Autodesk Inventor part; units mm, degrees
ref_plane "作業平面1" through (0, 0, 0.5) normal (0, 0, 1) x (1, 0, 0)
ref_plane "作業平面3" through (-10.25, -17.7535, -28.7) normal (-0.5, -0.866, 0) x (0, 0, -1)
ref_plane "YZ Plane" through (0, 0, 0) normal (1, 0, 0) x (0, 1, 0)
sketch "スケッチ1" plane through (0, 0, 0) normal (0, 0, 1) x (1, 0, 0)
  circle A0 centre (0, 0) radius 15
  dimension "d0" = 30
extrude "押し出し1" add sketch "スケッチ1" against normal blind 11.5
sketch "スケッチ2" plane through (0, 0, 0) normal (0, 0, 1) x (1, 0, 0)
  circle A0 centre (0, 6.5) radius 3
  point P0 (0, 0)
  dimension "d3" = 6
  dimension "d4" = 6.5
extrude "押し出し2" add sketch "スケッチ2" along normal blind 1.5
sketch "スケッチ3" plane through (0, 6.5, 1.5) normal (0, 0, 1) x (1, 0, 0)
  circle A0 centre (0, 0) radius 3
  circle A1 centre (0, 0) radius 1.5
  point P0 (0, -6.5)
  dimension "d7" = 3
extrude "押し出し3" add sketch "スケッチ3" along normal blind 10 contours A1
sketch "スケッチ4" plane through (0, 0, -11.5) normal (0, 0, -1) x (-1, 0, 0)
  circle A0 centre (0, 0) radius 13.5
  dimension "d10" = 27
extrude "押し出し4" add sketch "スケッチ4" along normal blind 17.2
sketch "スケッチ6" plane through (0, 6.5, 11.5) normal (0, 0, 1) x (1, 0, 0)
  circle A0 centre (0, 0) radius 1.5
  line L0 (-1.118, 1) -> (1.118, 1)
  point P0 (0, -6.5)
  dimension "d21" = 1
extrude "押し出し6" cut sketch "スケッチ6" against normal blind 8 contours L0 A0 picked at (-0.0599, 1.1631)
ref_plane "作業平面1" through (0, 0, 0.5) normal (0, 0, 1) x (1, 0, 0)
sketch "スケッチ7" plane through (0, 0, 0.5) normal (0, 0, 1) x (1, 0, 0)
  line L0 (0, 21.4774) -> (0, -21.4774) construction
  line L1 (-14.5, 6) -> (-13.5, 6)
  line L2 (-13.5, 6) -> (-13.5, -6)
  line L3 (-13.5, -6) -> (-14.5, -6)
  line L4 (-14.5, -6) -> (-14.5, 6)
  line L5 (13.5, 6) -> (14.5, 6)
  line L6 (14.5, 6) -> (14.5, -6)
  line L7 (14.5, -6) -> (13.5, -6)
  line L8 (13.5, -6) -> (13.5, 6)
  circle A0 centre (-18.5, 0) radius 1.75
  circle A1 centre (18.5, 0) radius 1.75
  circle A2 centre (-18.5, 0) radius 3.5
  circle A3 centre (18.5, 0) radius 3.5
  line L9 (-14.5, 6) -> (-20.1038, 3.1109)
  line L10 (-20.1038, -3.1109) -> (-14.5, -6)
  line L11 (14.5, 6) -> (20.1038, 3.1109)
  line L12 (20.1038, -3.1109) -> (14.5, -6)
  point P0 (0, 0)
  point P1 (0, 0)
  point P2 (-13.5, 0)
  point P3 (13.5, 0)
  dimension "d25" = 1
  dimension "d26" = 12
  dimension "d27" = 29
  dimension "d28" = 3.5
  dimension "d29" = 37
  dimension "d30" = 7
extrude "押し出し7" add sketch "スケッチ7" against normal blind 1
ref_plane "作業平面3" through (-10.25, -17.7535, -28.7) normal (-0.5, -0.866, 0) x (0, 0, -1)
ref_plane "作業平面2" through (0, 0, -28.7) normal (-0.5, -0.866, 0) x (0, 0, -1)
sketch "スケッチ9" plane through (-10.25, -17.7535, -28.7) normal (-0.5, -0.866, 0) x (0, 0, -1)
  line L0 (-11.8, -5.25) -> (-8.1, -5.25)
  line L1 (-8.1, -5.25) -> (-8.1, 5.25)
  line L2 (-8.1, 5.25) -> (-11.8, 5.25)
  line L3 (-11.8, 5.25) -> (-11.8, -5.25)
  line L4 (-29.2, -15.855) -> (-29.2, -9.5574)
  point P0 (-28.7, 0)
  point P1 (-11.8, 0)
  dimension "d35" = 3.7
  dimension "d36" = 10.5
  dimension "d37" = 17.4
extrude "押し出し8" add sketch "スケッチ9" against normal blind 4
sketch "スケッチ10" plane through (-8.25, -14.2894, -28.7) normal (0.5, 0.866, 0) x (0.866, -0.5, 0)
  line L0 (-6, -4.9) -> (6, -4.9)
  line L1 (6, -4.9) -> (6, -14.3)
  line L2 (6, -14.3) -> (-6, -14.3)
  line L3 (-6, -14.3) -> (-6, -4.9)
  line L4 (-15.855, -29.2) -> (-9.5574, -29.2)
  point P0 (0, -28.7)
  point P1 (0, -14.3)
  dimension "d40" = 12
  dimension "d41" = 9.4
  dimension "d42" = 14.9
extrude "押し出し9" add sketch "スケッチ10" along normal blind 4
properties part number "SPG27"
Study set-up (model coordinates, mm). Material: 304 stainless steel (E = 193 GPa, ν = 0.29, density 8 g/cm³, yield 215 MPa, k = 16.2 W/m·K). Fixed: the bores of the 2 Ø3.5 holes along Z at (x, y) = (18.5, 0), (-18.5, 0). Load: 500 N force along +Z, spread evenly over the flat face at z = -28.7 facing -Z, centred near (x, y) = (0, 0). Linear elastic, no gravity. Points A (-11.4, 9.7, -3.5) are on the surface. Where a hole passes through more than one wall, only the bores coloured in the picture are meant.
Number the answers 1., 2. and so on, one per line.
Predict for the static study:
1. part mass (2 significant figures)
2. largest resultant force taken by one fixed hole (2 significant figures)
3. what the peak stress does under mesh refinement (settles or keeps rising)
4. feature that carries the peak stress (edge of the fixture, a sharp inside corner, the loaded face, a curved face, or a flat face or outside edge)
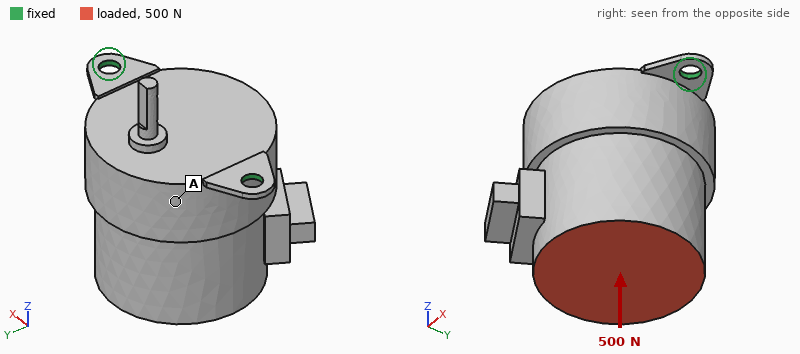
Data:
1. 150 g
2. 310 N
3. keeps rising
4. edge of the fixture
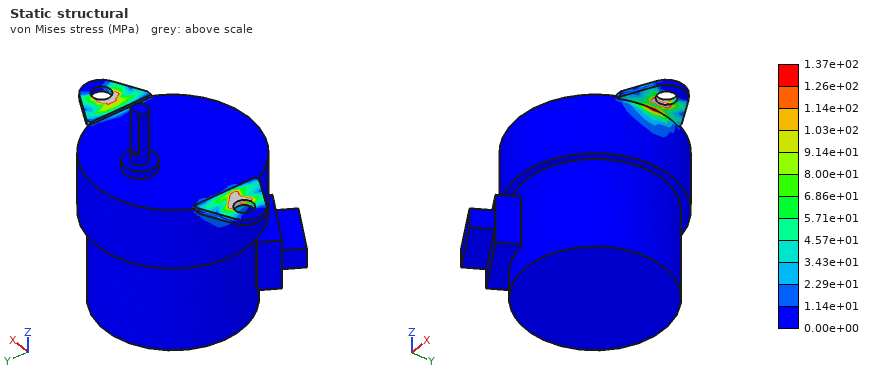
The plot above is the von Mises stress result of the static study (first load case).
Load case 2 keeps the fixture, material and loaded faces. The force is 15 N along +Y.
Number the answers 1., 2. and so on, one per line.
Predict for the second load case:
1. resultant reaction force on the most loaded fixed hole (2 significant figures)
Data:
1. 7.5 N
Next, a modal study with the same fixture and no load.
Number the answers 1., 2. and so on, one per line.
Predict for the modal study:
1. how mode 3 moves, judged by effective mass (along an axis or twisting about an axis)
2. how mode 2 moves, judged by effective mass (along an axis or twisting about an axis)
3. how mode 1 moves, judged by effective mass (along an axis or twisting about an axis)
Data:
1. along Z
2. along X
3. along Y
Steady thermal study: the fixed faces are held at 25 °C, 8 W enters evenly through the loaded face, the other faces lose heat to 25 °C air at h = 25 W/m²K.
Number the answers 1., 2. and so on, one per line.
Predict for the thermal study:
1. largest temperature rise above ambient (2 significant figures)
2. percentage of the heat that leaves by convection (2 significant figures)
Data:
1. 64 K
2. 61 %
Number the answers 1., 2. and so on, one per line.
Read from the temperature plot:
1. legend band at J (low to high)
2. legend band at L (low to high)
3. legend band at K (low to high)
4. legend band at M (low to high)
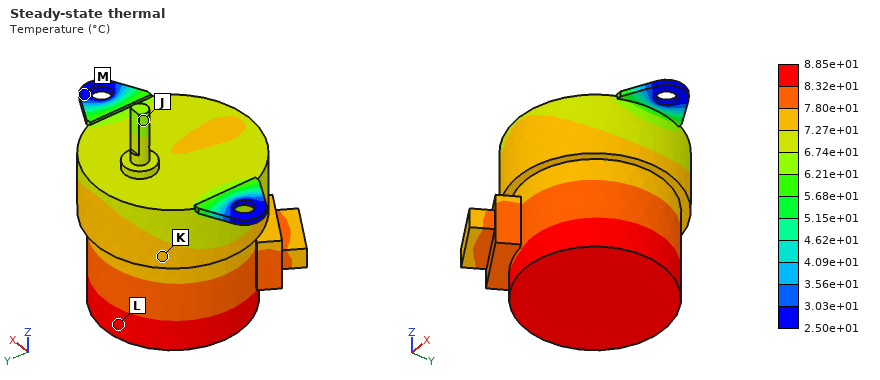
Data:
1. 6.21e+01 to 6.74e+01 °C
2. 8.32e+01 to 8.85e+01 °C
3. 7.27e+01 to 7.80e+01 °C
4. 2.50e+01 to 3.03e+01 °C
